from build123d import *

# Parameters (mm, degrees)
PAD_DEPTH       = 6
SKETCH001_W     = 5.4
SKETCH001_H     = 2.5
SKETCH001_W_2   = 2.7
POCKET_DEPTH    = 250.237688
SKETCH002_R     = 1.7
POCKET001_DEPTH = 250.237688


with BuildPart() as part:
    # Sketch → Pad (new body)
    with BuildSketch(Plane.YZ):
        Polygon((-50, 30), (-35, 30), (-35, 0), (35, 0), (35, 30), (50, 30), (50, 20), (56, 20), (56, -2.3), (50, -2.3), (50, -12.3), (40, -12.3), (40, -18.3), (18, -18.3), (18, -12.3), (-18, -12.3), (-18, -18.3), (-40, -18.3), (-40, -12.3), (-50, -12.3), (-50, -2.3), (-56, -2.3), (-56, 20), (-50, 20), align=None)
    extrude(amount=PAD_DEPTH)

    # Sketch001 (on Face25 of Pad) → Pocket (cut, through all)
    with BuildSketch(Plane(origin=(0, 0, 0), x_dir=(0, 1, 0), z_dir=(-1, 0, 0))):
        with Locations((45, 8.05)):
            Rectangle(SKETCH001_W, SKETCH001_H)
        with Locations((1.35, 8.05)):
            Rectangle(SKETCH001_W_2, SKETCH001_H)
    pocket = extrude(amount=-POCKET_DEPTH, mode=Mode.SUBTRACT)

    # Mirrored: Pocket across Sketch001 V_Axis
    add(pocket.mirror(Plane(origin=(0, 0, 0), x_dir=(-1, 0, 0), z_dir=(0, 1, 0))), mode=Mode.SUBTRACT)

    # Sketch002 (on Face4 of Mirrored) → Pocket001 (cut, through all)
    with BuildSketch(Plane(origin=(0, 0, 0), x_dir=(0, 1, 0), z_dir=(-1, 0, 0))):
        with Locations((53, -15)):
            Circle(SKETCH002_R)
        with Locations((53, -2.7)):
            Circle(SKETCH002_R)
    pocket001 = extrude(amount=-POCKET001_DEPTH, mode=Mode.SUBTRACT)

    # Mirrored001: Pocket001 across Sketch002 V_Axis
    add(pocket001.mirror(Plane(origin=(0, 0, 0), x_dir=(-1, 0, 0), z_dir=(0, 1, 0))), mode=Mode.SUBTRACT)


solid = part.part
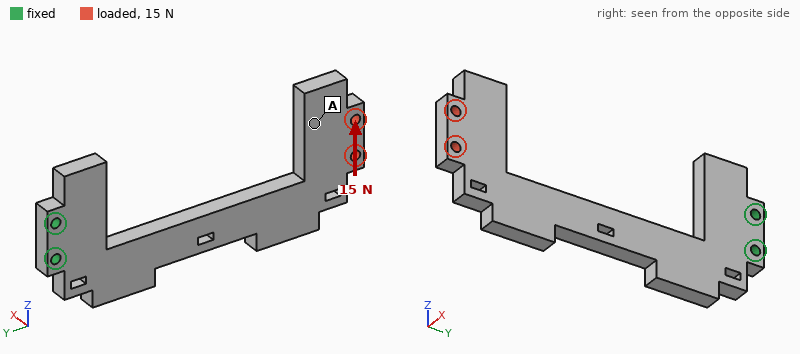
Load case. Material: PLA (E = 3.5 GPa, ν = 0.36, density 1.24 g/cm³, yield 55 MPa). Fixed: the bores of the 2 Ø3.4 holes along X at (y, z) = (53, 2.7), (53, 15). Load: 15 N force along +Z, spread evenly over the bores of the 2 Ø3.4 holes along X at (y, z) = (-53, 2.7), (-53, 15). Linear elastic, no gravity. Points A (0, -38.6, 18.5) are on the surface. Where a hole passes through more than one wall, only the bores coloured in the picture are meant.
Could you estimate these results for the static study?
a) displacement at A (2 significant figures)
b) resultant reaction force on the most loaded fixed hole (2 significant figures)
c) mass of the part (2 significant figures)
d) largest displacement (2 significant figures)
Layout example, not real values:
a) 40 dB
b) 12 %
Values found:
a) 1.1 mm
b) 120 N
c) 19 g
d) 1.4 mm
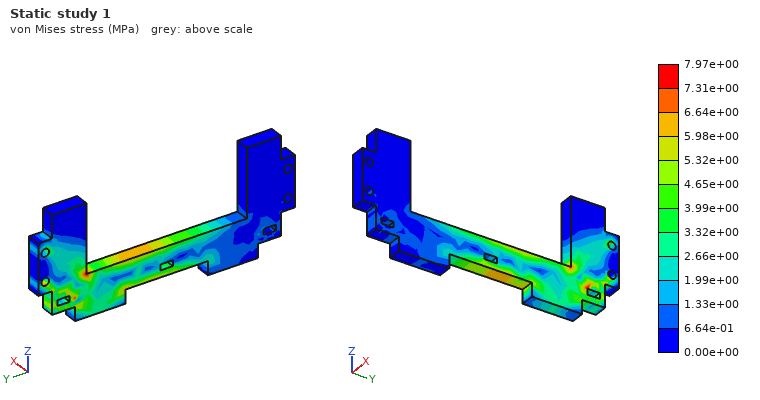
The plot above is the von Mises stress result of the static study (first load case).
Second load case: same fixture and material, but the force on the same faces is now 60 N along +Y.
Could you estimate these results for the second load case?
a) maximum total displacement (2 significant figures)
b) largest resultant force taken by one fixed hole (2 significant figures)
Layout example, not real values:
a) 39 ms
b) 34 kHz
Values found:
a) 1.2 mm
b) 33 N
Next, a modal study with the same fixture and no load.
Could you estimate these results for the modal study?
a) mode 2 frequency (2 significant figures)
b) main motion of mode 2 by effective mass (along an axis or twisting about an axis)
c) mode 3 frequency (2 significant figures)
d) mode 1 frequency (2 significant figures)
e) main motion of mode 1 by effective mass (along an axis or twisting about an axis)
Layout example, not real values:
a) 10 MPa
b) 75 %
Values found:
a) 220 Hz
b) along Z
c) 410 Hz
d) 99 Hz
e) along X
